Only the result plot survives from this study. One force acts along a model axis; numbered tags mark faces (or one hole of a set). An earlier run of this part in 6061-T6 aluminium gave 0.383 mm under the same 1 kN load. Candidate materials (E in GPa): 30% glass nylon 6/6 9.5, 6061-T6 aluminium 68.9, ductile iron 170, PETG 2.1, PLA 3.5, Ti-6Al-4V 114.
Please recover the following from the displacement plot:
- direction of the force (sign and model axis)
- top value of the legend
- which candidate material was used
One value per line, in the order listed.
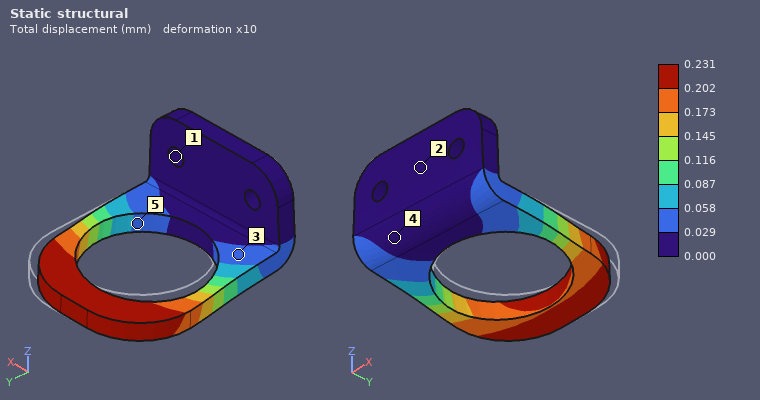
-X
0.231 mm
Ti-6Al-4V
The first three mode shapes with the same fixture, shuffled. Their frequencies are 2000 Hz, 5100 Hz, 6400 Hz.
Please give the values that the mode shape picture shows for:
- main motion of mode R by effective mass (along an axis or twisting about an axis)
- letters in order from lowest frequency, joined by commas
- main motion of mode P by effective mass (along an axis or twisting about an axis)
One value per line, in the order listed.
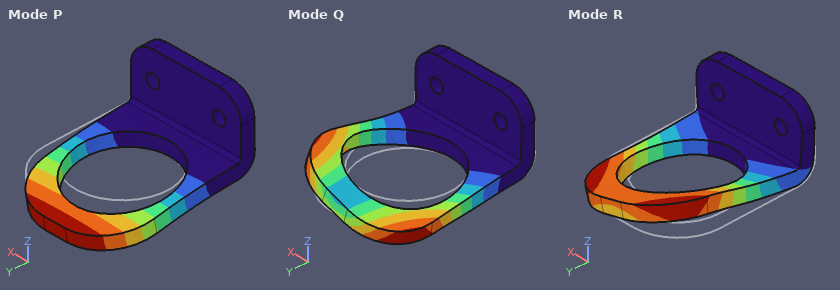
along X
P, R, Q
along Z
